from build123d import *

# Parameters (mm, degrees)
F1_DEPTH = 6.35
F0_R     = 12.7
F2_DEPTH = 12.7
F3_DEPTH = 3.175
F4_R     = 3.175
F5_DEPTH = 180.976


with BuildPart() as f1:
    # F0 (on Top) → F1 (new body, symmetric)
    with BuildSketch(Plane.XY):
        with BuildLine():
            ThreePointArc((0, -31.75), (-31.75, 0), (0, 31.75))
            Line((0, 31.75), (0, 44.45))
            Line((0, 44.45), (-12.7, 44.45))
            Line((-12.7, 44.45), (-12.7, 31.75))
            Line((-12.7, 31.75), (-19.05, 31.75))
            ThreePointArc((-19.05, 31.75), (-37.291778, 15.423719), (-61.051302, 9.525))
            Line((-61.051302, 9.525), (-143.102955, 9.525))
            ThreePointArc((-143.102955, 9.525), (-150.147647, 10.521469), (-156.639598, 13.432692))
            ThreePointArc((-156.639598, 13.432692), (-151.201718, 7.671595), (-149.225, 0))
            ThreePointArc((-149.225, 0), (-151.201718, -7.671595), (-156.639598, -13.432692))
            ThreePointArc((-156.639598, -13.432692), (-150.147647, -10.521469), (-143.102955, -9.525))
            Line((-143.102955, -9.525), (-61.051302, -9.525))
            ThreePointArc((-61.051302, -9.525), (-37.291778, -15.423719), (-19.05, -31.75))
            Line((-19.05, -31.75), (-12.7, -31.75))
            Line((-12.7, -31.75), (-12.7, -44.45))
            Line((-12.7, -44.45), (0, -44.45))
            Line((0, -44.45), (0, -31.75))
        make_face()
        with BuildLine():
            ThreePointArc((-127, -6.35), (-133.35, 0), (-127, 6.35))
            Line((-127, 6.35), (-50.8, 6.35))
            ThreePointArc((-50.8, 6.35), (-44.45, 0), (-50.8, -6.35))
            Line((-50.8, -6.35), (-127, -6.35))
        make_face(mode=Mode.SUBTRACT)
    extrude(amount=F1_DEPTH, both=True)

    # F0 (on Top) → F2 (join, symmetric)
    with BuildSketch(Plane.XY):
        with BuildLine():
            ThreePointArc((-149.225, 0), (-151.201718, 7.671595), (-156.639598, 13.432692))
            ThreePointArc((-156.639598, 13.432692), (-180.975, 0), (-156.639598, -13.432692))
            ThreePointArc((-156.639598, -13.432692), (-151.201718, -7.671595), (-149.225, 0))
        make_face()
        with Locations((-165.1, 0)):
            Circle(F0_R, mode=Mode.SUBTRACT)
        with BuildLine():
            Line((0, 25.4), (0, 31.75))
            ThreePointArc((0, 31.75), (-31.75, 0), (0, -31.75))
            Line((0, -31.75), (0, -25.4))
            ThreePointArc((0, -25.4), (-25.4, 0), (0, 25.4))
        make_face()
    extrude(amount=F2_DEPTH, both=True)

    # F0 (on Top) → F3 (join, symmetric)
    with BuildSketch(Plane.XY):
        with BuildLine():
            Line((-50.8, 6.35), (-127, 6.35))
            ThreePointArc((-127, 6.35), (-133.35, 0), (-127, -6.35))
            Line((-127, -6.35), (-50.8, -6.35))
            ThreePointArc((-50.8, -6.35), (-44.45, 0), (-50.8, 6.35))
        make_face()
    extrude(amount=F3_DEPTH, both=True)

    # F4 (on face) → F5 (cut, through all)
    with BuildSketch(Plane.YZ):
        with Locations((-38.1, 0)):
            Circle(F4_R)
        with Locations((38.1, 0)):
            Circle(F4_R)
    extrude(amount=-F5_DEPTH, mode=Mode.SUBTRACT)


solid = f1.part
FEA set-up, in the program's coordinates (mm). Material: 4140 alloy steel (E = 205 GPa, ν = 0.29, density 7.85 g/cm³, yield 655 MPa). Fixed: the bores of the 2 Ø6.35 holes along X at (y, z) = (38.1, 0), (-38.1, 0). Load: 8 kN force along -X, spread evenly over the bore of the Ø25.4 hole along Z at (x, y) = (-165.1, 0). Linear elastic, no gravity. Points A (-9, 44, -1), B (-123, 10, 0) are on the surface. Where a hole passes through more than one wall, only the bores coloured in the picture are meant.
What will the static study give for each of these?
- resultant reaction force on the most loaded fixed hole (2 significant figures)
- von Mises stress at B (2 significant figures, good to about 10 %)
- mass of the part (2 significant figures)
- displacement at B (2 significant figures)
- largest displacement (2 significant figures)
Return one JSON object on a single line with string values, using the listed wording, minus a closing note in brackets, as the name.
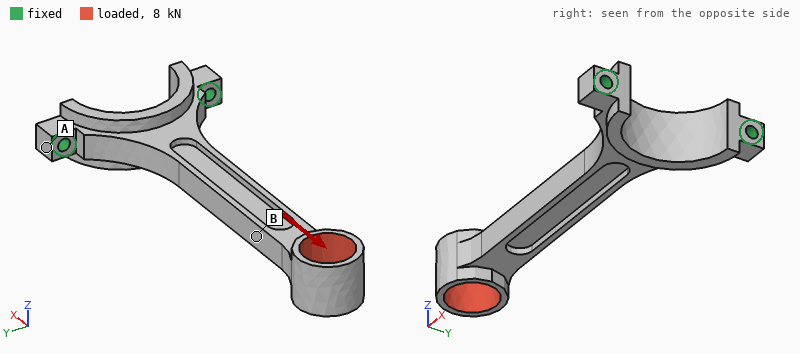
{"resultant reaction force on the most loaded fixed hole": "5.1 kN", "von Mises stress at B": "48 MPa", "mass of the part": "410 g", "displacement at B": "28 µm", "largest displacement": "73 µm"}
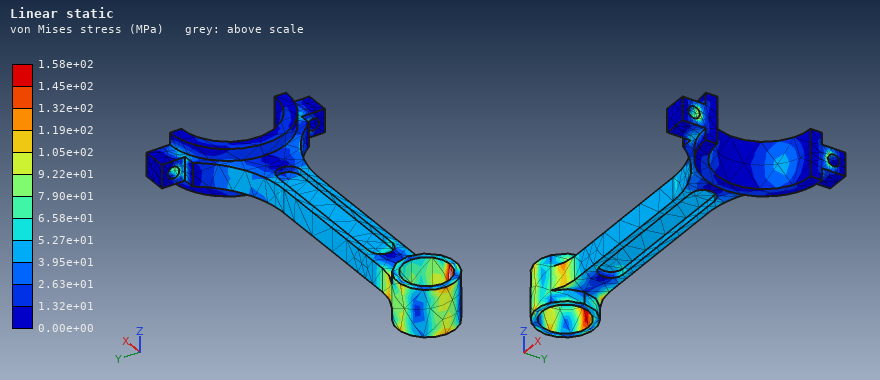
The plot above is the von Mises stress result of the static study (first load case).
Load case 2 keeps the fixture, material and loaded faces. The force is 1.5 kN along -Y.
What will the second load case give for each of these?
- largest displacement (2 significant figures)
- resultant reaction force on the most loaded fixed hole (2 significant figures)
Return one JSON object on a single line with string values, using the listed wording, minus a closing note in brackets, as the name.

{"largest displacement": "1.0 mm", "resultant reaction force on the most loaded fixed hole": "4.4 kN"}
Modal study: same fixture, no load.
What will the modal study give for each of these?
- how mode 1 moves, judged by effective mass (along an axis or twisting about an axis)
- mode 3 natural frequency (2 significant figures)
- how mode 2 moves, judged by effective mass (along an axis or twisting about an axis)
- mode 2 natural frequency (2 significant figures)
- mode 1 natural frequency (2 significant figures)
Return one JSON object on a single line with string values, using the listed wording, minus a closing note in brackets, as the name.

{"how mode 1 moves, judged by effective mass": "along Z", "mode 3 natural frequency": "1800 Hz", "how mode 2 moves, judged by effective mass": "along Y", "mode 2 natural frequency": "710 Hz", "mode 1 natural frequency": "310 Hz"}
